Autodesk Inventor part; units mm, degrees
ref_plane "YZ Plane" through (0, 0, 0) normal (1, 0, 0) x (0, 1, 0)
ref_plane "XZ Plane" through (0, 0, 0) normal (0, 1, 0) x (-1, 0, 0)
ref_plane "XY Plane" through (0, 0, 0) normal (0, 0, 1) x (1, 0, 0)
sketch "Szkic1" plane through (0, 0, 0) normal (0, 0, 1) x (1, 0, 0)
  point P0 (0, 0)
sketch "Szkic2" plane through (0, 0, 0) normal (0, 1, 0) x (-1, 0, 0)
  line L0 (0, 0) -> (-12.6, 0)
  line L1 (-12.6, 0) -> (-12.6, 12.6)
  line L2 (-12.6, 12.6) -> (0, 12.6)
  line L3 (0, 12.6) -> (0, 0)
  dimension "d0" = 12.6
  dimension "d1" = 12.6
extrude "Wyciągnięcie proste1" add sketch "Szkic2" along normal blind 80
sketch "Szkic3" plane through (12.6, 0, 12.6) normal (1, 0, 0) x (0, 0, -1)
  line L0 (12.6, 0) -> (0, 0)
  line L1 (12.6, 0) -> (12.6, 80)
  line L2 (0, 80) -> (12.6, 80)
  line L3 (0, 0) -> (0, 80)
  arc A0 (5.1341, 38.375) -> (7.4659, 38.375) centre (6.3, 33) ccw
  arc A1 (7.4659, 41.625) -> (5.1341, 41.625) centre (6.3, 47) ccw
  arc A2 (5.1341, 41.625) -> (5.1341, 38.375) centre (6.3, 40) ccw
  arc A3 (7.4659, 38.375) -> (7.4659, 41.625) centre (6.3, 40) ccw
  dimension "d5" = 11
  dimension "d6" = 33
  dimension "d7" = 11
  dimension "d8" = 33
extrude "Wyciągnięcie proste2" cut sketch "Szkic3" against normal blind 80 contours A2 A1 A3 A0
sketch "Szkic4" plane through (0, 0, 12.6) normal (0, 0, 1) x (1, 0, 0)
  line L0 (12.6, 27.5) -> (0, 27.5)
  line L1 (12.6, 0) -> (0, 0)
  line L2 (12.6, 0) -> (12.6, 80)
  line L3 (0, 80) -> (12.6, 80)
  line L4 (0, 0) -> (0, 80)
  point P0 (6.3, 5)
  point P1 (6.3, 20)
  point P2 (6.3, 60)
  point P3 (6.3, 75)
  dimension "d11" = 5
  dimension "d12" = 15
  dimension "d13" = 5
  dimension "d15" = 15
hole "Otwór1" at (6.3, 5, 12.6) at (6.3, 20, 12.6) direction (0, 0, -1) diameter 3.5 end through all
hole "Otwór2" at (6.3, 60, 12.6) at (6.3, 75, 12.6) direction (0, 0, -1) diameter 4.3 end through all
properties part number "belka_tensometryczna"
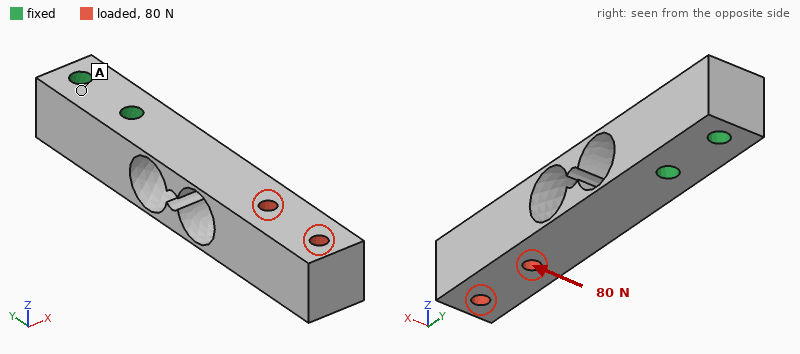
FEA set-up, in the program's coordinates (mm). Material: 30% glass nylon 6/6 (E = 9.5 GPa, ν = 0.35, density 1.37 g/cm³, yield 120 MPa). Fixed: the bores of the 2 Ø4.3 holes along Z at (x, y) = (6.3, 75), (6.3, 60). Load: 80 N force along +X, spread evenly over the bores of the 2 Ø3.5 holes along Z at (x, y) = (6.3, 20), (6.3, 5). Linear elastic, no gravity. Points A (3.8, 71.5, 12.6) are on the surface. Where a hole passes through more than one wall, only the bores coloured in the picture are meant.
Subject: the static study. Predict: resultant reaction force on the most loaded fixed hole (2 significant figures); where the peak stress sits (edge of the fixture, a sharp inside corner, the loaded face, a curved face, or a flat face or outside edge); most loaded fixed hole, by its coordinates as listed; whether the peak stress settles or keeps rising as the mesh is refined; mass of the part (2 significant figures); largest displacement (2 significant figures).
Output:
190 N
a sharp inside corner
(6.3, 60)
keeps rising
13 g
0.86 mm
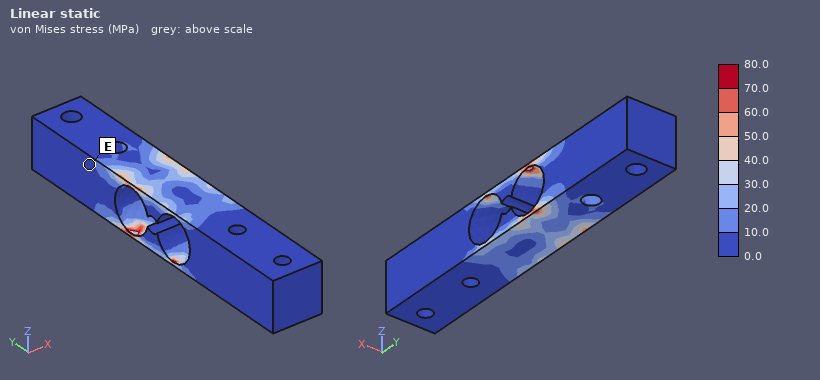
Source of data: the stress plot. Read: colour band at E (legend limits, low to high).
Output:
0.0 to 10.0 MPa
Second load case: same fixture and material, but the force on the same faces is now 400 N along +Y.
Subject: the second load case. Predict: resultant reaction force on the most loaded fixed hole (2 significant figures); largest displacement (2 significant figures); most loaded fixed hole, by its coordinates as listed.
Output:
360 N
51 µm
(6.3, 60)
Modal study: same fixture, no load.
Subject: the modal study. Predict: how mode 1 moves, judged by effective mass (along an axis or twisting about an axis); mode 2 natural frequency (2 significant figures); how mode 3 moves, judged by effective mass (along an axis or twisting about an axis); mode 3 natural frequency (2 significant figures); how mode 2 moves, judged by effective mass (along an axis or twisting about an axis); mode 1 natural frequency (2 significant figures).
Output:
along Z
760 Hz
twisting about Y
2600 Hz
along X
350 Hz
